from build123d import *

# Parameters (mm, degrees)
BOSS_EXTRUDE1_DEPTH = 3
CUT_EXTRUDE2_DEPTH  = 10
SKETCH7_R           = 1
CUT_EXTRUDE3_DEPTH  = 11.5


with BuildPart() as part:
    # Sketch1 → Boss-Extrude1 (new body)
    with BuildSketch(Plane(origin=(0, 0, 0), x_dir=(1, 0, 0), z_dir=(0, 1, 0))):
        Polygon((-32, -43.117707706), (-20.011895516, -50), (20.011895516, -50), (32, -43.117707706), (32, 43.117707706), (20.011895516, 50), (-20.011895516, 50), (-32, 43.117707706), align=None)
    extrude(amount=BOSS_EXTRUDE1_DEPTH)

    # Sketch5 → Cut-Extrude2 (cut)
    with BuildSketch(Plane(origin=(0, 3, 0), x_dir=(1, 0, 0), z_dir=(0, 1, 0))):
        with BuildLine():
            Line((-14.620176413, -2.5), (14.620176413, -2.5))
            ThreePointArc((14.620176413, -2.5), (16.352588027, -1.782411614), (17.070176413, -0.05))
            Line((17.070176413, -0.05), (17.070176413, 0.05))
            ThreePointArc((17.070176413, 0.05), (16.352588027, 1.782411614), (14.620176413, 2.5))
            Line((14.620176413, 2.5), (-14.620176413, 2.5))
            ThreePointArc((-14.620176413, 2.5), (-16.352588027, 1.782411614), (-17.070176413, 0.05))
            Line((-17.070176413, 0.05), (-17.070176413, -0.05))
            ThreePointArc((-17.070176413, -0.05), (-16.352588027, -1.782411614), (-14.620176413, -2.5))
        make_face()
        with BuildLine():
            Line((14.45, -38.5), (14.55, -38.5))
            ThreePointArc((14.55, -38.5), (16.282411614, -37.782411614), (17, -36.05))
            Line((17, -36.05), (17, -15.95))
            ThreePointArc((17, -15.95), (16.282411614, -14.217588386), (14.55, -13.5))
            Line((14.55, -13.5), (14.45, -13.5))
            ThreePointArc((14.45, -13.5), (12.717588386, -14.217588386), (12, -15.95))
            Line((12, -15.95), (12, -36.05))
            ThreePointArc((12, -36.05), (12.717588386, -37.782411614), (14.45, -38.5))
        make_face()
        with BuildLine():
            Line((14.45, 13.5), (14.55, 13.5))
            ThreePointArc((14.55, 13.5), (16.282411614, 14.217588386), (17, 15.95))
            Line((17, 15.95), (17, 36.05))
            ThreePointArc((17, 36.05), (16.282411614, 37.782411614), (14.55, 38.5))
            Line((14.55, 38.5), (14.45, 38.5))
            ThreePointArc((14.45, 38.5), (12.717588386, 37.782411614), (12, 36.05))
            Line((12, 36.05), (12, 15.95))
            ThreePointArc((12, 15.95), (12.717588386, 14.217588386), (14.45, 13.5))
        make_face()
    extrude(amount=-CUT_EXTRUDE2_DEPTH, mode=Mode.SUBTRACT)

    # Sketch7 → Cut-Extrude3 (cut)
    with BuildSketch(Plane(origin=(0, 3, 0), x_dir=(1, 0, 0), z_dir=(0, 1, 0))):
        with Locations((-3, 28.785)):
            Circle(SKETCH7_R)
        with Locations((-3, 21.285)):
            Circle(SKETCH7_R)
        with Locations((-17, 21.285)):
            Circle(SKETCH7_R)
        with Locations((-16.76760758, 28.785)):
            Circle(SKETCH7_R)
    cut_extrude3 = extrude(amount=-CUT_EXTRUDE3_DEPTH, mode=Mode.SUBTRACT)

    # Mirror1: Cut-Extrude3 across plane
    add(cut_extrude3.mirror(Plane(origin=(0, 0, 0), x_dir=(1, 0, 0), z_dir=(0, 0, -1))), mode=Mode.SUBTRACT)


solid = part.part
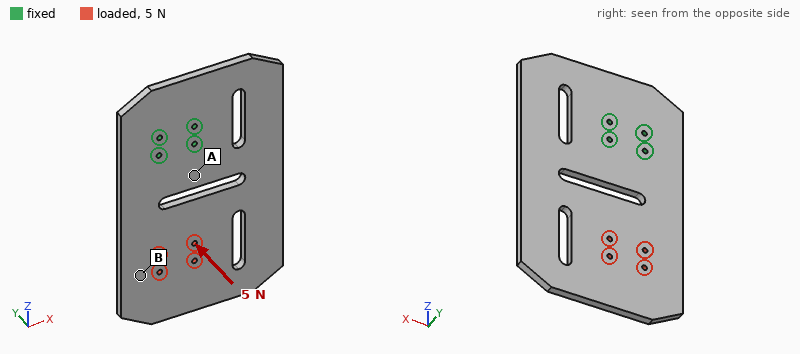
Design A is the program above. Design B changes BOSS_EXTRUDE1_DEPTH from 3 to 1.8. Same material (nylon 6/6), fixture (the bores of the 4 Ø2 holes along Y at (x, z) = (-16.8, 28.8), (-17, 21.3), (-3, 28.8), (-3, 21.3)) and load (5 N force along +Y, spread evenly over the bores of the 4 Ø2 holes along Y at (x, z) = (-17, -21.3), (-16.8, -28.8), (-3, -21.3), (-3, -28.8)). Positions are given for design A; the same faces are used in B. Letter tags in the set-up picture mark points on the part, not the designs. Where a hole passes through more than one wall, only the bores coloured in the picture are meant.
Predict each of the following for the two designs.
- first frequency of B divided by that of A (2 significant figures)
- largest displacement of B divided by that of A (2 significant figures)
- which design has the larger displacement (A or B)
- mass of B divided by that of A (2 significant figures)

0.61
4.5
B
0.60
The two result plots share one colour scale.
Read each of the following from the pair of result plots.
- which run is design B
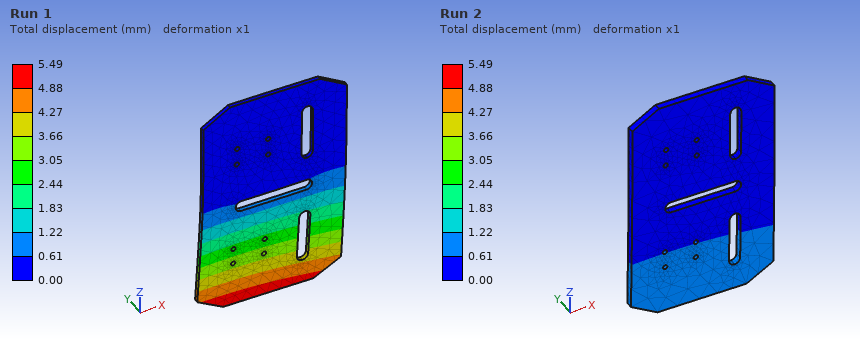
Run 1
